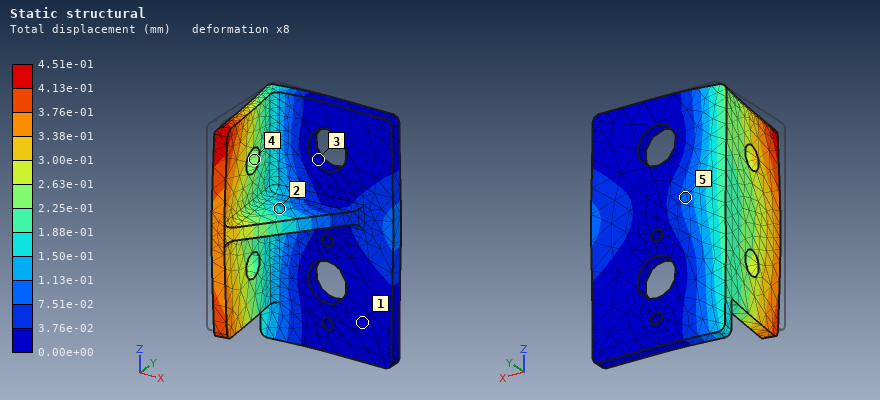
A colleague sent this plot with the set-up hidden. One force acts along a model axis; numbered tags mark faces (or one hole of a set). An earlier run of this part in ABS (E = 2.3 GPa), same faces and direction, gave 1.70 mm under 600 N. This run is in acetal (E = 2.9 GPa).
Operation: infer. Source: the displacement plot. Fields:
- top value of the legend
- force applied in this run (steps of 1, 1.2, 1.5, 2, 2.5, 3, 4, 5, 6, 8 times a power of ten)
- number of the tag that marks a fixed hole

4.51e-01 mm
200 N
3
